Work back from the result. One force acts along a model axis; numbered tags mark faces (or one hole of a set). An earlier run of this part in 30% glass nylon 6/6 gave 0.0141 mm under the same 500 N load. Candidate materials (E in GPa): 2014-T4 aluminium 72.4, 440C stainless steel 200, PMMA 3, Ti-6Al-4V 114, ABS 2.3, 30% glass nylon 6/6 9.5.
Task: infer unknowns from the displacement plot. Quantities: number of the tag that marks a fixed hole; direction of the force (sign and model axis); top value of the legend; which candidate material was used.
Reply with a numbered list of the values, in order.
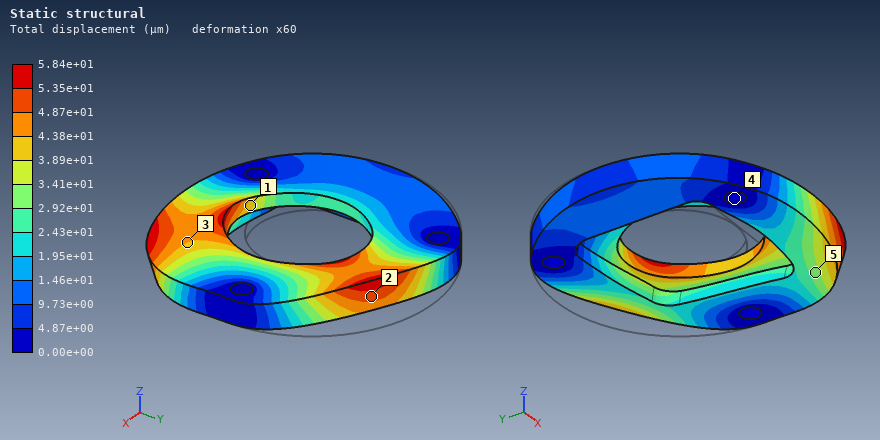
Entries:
1. 4
2. -Y
3. 5.84e+01 µm
4. ABS
